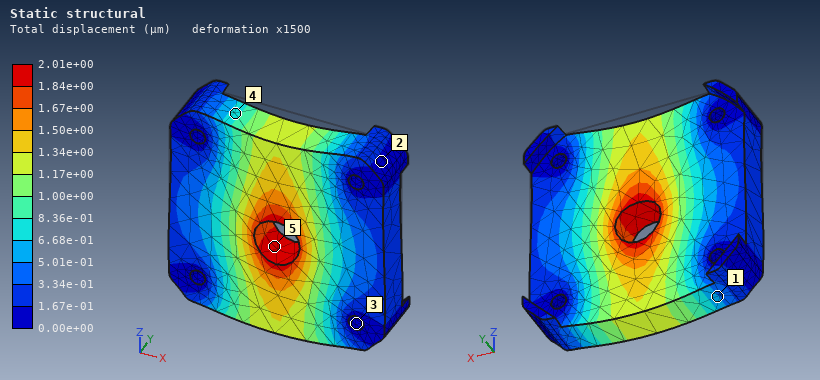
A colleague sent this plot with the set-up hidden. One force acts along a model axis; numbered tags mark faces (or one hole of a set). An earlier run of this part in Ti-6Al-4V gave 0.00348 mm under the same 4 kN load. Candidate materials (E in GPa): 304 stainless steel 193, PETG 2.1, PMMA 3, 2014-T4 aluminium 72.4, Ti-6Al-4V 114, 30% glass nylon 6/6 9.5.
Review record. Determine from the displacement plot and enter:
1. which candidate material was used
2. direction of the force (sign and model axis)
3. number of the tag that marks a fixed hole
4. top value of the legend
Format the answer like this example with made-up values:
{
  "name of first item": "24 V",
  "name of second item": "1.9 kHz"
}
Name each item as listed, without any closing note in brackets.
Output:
{
  "which candidate material was used": "304 stainless steel",
  "direction of the force": "-Z",
  "number of the tag that marks a fixed hole": "3",
  "top value of the legend": "2.01e+00 µm"
}
